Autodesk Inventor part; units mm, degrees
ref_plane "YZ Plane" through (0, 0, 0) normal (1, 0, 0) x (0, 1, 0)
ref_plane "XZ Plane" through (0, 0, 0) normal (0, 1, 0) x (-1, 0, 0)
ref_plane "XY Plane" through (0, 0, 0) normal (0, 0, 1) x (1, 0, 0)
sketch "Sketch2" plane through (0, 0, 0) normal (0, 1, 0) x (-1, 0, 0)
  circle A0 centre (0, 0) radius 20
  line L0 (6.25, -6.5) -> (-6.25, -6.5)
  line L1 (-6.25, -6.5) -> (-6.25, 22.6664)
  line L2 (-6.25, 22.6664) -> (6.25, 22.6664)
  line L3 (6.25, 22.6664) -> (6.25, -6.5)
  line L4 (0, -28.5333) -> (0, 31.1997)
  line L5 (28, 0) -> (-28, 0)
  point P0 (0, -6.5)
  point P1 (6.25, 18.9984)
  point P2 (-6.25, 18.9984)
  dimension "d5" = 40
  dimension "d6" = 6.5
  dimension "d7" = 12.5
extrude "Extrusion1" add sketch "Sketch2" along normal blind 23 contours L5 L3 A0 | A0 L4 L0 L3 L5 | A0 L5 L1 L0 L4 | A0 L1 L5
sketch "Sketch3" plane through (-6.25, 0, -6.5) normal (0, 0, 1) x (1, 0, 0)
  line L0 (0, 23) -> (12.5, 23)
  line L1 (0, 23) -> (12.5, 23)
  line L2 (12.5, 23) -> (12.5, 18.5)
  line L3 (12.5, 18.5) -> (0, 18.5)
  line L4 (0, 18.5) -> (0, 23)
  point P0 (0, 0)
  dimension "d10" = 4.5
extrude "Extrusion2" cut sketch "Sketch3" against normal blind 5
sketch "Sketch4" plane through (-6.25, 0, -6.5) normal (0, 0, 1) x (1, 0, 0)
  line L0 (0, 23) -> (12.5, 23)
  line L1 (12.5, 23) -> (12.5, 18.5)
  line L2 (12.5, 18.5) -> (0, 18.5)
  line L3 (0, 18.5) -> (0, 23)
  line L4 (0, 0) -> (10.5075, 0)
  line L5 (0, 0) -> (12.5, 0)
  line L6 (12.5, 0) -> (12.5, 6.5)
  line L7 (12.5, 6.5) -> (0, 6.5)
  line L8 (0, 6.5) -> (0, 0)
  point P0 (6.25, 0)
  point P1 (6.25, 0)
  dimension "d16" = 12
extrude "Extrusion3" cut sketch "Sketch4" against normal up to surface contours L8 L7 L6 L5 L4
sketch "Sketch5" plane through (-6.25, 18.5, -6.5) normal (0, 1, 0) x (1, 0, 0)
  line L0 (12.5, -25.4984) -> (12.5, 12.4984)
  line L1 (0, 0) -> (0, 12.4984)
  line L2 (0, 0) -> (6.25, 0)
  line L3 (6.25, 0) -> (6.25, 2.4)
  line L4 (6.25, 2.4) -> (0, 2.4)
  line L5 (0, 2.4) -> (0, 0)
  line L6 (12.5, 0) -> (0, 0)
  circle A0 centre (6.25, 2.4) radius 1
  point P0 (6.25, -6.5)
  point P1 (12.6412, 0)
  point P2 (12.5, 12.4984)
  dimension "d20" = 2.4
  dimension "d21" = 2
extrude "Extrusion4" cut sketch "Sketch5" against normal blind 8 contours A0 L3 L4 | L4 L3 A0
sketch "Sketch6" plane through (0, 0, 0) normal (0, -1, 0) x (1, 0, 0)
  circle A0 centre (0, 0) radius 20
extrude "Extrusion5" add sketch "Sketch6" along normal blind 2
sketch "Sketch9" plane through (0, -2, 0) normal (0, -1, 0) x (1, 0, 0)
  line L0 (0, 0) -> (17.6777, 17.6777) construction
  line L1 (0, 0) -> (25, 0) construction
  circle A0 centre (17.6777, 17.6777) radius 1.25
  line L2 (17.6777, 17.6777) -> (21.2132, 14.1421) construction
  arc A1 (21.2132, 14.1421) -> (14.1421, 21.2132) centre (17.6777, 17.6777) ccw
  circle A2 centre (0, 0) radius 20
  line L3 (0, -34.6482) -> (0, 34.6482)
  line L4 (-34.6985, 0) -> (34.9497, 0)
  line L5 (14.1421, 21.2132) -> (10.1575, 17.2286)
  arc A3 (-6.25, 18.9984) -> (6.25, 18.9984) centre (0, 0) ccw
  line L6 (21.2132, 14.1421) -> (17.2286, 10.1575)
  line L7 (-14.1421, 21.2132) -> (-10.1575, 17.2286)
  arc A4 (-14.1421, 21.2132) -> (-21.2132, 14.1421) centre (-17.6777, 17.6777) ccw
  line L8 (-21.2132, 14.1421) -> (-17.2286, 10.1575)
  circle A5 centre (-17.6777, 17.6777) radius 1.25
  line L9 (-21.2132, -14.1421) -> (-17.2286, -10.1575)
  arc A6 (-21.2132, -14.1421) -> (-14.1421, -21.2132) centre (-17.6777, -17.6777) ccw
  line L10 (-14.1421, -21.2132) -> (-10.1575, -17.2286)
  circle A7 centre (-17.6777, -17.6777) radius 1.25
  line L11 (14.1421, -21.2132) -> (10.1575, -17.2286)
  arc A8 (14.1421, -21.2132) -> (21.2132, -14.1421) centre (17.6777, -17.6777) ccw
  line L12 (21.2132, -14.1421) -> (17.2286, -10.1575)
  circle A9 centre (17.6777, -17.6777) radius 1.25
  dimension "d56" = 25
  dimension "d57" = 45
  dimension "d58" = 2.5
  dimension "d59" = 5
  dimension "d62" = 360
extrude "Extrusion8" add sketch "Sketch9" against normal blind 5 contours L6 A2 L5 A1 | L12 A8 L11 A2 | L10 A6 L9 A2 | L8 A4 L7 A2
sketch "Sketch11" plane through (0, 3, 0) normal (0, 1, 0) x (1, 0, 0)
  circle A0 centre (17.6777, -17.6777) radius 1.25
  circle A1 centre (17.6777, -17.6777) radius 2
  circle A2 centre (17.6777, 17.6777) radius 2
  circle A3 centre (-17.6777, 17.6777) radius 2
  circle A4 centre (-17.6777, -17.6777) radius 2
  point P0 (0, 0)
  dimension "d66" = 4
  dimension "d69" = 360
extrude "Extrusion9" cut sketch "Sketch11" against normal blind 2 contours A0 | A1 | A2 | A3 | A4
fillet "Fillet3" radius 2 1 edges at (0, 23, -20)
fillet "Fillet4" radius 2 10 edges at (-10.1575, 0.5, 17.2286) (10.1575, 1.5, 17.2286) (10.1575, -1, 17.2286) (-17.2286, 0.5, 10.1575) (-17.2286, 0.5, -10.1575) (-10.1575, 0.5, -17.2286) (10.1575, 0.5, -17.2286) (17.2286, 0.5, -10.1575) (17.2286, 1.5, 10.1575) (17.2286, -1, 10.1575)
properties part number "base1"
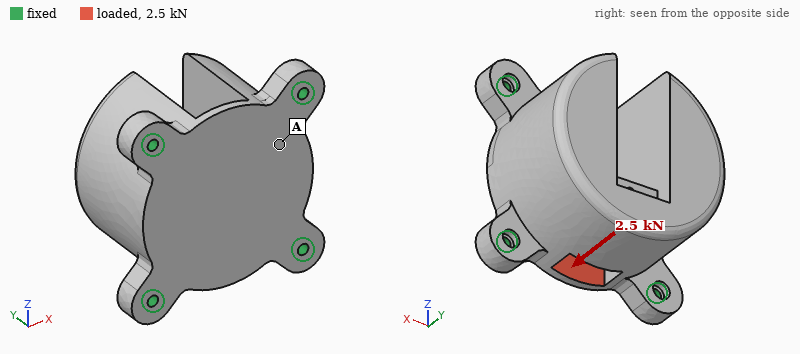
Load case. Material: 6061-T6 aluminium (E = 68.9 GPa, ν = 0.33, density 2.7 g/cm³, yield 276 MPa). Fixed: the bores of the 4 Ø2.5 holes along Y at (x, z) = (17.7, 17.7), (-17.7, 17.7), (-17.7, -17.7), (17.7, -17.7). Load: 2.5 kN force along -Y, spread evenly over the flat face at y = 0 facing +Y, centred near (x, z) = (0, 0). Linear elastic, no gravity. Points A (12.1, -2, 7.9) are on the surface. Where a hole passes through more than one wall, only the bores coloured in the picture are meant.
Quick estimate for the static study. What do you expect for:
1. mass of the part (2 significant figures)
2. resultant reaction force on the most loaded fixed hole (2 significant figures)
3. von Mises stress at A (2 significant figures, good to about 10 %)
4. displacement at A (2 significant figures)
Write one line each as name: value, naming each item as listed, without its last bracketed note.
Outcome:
mass of the part: 65 g
resultant reaction force on the most loaded fixed hole: 780 N
von Mises stress at A: 18 MPa
displacement at A: 12 µm
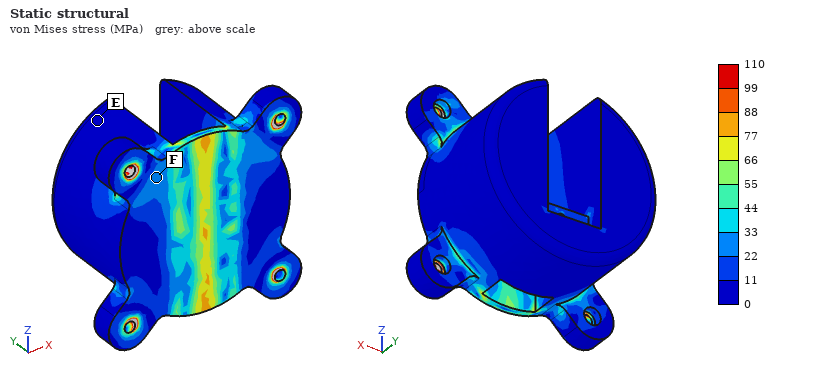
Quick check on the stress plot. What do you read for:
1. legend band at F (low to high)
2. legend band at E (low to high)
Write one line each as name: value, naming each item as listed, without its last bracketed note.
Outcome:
legend band at F: 22 to 33 MPa
legend band at E: 0 to 11 MPa
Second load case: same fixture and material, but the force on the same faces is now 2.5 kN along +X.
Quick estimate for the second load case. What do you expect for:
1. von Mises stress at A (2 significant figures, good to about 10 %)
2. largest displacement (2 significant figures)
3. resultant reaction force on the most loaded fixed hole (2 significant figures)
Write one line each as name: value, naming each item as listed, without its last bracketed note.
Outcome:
von Mises stress at A: 8.5 MPa
largest displacement: 6.4 µm
resultant reaction force on the most loaded fixed hole: 690 N
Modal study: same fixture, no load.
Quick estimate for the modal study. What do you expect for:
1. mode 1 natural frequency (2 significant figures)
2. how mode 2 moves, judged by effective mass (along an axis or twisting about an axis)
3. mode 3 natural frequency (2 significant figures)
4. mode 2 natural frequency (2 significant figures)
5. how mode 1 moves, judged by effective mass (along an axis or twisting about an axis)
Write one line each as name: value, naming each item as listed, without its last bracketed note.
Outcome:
mode 1 natural frequency: 8300 Hz
how mode 2 moves, judged by effective mass: along Y
mode 3 natural frequency: 10 kHz
mode 2 natural frequency: 9600 Hz
how mode 1 moves, judged by effective mass: along X
